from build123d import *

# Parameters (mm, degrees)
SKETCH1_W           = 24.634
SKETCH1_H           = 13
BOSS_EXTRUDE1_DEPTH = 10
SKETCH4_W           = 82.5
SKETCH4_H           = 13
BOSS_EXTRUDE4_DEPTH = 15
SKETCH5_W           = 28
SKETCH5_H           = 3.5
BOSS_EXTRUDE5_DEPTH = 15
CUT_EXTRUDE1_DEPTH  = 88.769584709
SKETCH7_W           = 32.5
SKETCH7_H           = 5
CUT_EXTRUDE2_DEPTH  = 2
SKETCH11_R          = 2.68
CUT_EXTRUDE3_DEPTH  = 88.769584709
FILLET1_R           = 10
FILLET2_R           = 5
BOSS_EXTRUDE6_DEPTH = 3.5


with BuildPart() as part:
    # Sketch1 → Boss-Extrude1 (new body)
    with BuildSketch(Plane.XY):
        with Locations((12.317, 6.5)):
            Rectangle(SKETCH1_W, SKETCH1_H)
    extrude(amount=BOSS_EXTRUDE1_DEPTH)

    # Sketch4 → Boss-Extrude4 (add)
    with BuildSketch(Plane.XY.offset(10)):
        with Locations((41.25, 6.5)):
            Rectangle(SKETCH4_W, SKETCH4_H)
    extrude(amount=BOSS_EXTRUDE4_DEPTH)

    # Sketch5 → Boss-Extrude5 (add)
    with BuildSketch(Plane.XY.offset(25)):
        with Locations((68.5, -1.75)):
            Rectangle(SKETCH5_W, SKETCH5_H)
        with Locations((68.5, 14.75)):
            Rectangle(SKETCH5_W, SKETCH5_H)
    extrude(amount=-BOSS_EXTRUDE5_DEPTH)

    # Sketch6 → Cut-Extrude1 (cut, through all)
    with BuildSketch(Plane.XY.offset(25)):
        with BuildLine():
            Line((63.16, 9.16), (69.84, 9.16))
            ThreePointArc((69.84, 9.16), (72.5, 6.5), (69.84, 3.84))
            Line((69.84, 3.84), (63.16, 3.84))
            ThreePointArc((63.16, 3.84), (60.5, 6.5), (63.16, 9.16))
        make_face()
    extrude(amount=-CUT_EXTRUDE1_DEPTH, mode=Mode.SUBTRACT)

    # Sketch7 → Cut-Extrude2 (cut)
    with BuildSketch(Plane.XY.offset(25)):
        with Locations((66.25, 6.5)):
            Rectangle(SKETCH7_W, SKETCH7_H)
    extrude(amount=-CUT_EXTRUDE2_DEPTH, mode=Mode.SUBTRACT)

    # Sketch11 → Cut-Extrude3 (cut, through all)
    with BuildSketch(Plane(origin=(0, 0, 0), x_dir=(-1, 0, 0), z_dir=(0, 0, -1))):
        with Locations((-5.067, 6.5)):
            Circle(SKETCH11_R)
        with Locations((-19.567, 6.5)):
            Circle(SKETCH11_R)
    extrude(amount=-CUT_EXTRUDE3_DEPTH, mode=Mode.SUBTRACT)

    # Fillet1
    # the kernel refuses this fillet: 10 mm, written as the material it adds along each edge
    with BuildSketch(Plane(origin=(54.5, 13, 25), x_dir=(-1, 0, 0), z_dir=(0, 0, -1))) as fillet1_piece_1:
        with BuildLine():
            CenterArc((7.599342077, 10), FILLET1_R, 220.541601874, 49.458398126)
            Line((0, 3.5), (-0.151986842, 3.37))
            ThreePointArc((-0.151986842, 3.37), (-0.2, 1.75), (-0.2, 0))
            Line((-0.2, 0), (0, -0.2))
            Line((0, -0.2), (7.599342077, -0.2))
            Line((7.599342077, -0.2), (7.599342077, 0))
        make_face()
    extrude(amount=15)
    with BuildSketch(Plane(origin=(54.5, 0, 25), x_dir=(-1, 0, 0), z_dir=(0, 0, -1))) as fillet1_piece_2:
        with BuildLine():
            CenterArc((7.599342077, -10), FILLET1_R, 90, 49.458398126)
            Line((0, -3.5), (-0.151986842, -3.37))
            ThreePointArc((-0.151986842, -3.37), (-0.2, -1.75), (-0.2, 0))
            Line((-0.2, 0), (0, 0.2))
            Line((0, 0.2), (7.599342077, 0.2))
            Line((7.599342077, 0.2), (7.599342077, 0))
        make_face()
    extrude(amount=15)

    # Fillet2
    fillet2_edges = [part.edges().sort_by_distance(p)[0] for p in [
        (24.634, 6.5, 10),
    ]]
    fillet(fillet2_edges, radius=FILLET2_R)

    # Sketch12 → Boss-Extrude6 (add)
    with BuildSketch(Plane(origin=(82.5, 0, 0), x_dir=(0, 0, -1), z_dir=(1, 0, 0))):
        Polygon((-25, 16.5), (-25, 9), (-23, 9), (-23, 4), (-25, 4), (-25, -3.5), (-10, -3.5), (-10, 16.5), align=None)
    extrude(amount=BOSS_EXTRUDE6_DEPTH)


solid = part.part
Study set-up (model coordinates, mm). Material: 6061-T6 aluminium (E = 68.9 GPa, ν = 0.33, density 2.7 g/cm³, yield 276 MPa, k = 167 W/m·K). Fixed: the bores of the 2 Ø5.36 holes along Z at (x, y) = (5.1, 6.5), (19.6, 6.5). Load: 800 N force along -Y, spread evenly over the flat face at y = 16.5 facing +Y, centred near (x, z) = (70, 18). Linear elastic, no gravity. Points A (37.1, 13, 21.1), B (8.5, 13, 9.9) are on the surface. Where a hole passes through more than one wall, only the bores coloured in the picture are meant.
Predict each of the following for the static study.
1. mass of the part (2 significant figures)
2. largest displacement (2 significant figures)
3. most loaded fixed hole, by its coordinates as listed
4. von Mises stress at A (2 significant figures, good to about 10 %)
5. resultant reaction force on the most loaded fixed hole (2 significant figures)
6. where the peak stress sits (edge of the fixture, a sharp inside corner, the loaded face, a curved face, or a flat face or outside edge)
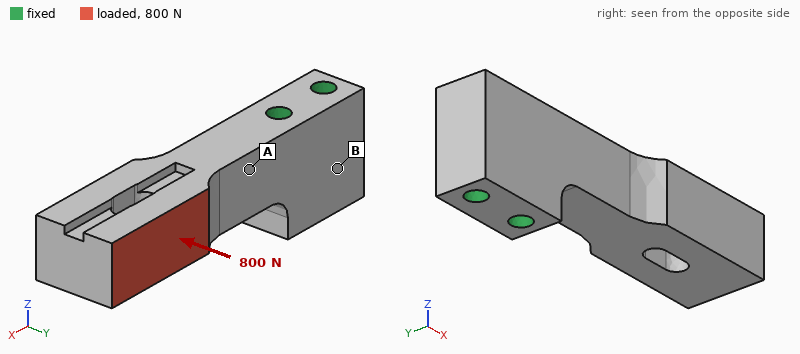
58 g
0.28 mm
(19.6, 6.5)
62 MPa
1.7 kN
a curved face
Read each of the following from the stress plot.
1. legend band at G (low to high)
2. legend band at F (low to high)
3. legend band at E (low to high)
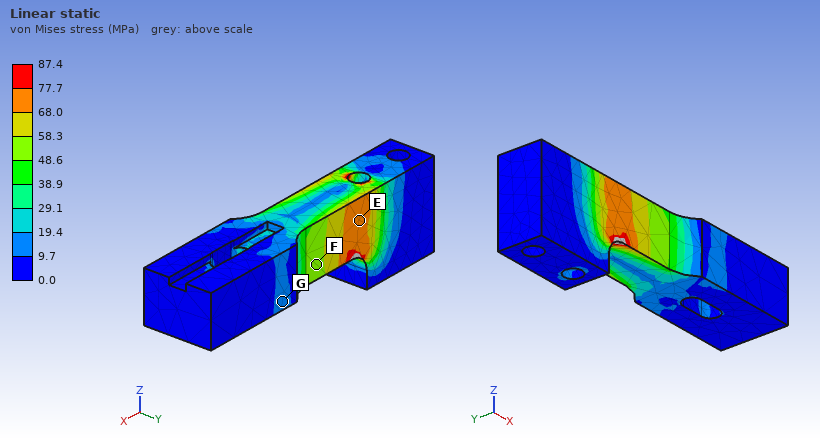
9.7 to 19.4 MPa
48.6 to 58.3 MPa
68.0 to 77.7 MPa
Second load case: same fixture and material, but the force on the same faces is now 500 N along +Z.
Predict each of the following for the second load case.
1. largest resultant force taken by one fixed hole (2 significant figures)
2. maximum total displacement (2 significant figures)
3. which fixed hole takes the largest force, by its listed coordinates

560 N
0.13 mm
(19.6, 6.5)
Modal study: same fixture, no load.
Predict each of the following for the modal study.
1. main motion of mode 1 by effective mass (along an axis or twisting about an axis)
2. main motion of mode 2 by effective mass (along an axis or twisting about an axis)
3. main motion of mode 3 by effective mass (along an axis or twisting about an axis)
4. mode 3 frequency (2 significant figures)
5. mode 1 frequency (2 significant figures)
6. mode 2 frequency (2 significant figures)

along Y
along Z
twisting about X
8000 Hz
2000 Hz
2500 Hz
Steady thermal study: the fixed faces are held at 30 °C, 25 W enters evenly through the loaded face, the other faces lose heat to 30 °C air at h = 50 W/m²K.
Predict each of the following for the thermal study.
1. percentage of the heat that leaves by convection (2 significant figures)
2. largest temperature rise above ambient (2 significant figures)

17 %
32 K
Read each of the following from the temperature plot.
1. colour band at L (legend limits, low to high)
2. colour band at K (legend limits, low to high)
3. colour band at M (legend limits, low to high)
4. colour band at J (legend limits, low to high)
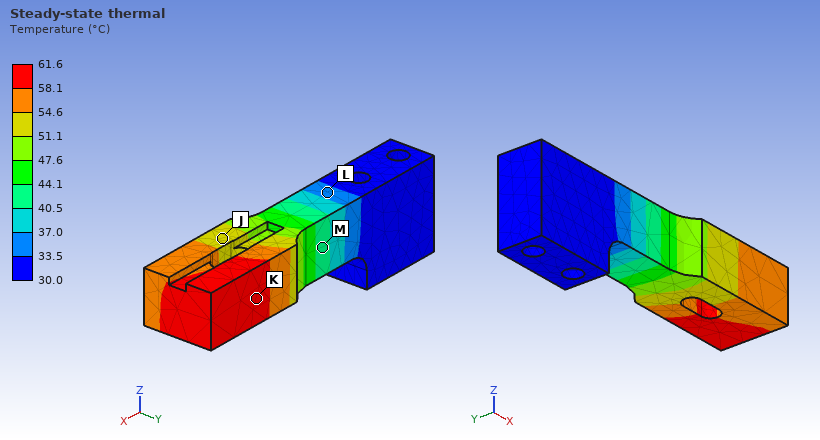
33.5 to 37.0 °C
58.1 to 61.6 °C
40.5 to 44.1 °C
51.1 to 54.6 °C
